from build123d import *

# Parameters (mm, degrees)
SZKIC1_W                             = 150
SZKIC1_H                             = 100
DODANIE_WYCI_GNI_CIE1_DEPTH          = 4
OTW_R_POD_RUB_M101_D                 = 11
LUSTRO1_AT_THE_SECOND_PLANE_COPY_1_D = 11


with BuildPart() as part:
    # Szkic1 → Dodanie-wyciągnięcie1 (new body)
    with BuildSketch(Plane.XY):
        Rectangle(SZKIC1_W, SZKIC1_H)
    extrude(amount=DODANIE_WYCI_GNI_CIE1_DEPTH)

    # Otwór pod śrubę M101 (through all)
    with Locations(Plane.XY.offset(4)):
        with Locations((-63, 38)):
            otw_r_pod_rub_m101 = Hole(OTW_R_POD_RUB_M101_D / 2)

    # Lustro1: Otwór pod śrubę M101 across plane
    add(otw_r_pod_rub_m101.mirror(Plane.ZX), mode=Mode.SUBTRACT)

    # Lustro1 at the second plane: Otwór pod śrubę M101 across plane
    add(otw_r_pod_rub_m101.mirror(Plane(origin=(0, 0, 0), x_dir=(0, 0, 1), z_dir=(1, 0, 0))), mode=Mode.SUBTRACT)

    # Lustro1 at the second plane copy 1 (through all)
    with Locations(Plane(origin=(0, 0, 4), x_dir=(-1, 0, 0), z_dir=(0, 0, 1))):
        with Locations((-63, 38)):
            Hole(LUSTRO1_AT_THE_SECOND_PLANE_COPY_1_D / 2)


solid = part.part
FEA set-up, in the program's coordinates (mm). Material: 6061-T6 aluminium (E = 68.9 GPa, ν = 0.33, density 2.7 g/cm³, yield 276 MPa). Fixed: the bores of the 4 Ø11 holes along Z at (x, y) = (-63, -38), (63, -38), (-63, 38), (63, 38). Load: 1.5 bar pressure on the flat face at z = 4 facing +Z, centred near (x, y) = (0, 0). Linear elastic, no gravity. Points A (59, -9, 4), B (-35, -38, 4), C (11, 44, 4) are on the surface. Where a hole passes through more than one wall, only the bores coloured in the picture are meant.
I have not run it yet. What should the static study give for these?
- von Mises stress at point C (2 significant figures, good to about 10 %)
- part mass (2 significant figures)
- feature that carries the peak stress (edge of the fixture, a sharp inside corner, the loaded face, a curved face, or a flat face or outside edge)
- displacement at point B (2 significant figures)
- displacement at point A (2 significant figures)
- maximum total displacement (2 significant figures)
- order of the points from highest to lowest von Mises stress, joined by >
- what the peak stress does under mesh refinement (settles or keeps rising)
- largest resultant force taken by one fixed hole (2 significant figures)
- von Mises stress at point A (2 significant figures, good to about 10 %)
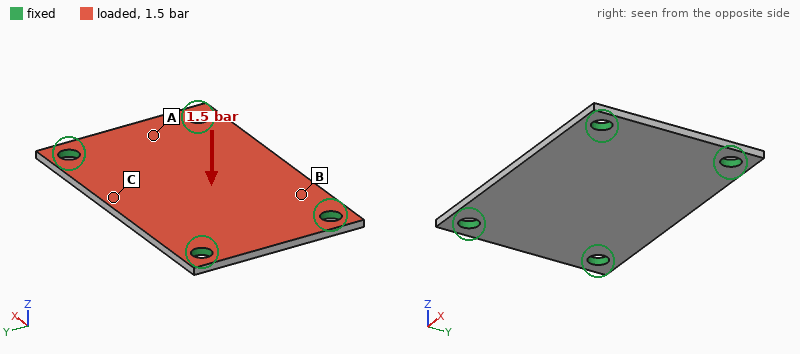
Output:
35 MPa
160 g
edge of the fixture
0.12 mm
0.045 mm
0.27 mm
C > A > B
keeps rising
550 N
21 MPa
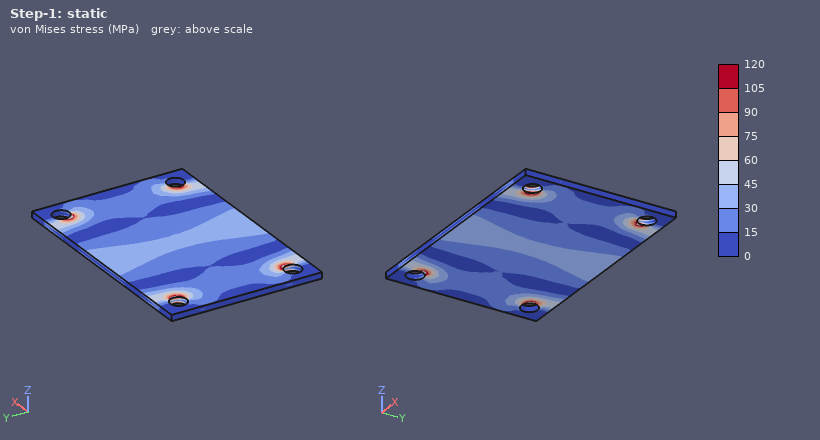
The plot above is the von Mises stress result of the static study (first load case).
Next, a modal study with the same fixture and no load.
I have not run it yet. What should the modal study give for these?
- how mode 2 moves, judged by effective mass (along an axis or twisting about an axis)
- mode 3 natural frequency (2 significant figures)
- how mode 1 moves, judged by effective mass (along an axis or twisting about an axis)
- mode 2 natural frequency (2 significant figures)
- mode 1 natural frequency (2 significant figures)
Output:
twisting about X
3100 Hz
along Z
1900 Hz
1300 Hz
